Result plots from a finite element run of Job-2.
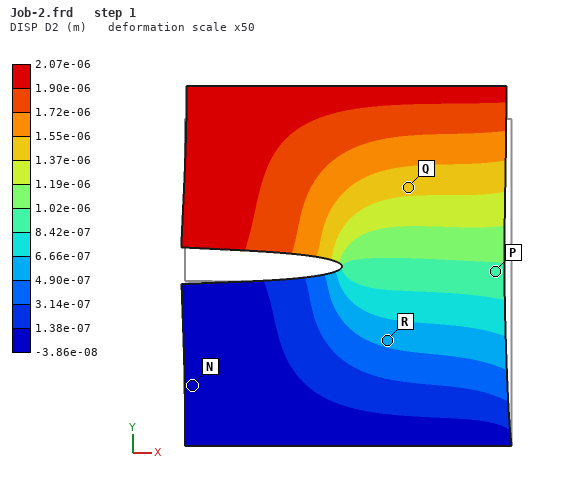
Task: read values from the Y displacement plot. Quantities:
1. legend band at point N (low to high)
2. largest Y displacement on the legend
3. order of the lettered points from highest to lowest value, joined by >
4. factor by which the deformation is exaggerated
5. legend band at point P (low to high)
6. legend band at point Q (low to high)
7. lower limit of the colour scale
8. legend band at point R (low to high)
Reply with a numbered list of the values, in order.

1. -3.86e-08 to 1.38e-07 m
2. 2.07e-06 m
3. Q > P > R > N
4. 50
5. 8.42e-07 to 1.02e-06 m
6. 1.37e-06 to 1.55e-06 m
7. -3.86e-08 m
8. 4.90e-07 to 6.66e-07 m
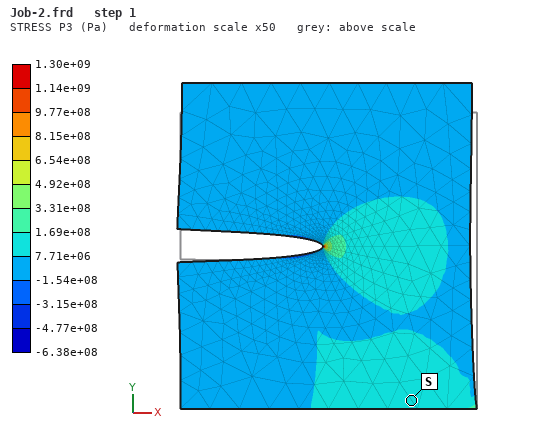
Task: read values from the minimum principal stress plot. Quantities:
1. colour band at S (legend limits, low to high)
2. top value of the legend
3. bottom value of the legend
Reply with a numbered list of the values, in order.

1. 7.71e+06 to 1.69e+08 Pa
2. 1.30e+09 Pa
3. -6.38e+08 Pa
